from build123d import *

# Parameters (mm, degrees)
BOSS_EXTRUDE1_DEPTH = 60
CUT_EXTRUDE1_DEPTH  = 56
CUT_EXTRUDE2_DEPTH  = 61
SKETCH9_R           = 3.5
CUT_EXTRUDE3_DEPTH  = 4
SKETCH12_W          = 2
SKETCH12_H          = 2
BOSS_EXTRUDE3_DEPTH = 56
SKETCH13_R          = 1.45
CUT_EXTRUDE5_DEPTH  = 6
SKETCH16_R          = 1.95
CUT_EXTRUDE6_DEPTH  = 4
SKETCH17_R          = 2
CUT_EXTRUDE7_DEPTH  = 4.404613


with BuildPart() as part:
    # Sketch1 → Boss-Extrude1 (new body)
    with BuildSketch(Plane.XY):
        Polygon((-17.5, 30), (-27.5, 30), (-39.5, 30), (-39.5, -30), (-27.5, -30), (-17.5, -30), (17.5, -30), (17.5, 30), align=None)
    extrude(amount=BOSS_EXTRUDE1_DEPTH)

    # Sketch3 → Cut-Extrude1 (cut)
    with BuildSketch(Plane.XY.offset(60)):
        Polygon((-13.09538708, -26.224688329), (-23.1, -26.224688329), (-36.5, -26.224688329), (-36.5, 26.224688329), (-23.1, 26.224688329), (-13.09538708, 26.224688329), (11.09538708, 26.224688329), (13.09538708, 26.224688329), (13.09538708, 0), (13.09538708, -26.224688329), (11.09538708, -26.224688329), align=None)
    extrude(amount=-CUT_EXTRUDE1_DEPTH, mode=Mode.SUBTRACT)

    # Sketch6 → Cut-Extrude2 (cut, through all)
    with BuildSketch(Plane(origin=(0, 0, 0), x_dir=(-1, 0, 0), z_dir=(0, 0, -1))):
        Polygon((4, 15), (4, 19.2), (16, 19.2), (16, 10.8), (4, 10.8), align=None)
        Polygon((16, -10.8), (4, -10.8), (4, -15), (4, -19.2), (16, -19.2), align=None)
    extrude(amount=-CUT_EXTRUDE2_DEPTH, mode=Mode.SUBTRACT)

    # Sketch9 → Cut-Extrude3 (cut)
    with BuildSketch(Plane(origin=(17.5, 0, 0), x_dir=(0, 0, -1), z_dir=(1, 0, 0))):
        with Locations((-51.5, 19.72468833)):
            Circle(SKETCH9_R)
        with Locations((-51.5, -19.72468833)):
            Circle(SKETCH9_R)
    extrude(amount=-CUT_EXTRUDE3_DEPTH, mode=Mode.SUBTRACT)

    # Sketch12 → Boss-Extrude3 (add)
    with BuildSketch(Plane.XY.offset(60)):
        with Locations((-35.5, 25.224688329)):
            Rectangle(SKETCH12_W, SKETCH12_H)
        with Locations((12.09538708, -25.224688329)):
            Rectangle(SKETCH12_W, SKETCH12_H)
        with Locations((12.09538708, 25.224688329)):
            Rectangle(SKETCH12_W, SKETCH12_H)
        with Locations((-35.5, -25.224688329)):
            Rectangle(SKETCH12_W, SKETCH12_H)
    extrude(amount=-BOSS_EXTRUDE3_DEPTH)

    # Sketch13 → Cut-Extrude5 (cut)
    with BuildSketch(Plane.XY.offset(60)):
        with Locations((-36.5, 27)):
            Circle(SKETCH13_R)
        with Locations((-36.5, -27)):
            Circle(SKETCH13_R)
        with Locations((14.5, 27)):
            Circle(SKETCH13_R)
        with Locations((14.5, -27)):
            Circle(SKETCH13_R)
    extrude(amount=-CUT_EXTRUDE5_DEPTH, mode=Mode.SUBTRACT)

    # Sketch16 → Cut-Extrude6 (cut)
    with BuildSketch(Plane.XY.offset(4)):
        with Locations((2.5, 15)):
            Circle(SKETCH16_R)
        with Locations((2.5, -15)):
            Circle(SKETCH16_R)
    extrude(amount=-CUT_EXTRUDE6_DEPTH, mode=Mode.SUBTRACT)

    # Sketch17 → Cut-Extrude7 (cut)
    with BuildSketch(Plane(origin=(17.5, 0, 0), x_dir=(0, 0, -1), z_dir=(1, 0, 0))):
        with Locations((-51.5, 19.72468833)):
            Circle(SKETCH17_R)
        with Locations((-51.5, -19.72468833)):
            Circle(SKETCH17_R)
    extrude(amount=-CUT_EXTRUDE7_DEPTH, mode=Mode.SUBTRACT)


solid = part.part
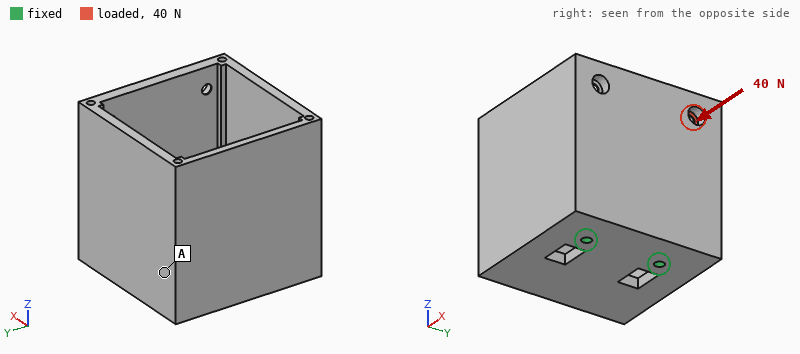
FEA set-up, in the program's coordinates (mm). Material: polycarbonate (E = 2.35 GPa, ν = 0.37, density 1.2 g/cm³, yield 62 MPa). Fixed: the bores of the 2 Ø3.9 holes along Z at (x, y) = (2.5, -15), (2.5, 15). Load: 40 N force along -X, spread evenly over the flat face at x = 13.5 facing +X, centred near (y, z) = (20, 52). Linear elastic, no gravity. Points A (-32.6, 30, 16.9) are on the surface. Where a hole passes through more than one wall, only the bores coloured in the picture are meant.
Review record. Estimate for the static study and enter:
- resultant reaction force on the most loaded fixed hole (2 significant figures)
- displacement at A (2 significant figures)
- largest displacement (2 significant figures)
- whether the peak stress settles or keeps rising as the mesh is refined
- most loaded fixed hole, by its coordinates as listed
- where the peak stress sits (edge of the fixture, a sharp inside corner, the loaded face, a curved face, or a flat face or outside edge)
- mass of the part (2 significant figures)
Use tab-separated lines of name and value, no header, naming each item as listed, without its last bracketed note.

resultant reaction force on the most loaded fixed hole	45 N
displacement at A	0.67 mm
largest displacement	1.2 mm
whether the peak stress settles or keeps rising as the mesh is refined	keeps rising
most loaded fixed hole, by its coordinates as listed	(2.5, 15)
where the peak stress sits	edge of the fixture
mass of the part	71 g
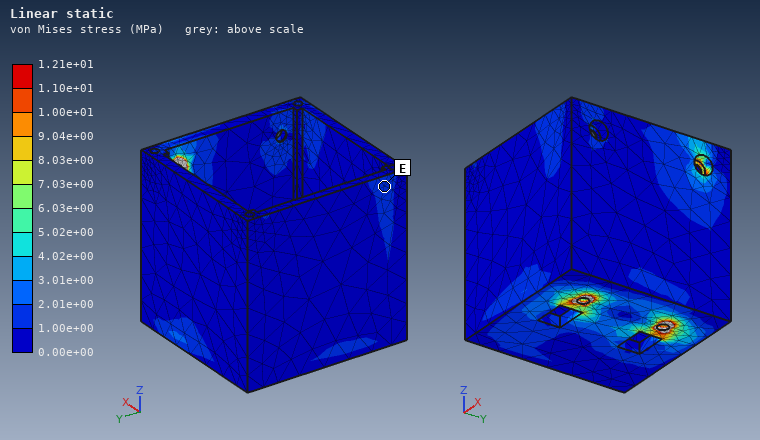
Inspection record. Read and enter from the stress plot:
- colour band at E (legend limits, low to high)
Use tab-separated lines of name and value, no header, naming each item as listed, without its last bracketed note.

colour band at E	1.00e+00 to 2.01e+00 MPa
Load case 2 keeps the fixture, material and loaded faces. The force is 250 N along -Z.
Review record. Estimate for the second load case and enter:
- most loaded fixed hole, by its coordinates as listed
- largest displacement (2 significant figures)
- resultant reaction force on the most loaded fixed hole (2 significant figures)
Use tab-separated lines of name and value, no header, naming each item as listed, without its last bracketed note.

most loaded fixed hole, by its coordinates as listed	(2.5, 15)
largest displacement	1.2 mm
resultant reaction force on the most loaded fixed hole	260 N
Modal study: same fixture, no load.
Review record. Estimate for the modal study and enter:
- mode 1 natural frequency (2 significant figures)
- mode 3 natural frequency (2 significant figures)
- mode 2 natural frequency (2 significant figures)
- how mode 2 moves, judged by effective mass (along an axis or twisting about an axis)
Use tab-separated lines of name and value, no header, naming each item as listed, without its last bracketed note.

mode 1 natural frequency	170 Hz
mode 3 natural frequency	640 Hz
mode 2 natural frequency	440 Hz
how mode 2 moves, judged by effective mass	along Y
